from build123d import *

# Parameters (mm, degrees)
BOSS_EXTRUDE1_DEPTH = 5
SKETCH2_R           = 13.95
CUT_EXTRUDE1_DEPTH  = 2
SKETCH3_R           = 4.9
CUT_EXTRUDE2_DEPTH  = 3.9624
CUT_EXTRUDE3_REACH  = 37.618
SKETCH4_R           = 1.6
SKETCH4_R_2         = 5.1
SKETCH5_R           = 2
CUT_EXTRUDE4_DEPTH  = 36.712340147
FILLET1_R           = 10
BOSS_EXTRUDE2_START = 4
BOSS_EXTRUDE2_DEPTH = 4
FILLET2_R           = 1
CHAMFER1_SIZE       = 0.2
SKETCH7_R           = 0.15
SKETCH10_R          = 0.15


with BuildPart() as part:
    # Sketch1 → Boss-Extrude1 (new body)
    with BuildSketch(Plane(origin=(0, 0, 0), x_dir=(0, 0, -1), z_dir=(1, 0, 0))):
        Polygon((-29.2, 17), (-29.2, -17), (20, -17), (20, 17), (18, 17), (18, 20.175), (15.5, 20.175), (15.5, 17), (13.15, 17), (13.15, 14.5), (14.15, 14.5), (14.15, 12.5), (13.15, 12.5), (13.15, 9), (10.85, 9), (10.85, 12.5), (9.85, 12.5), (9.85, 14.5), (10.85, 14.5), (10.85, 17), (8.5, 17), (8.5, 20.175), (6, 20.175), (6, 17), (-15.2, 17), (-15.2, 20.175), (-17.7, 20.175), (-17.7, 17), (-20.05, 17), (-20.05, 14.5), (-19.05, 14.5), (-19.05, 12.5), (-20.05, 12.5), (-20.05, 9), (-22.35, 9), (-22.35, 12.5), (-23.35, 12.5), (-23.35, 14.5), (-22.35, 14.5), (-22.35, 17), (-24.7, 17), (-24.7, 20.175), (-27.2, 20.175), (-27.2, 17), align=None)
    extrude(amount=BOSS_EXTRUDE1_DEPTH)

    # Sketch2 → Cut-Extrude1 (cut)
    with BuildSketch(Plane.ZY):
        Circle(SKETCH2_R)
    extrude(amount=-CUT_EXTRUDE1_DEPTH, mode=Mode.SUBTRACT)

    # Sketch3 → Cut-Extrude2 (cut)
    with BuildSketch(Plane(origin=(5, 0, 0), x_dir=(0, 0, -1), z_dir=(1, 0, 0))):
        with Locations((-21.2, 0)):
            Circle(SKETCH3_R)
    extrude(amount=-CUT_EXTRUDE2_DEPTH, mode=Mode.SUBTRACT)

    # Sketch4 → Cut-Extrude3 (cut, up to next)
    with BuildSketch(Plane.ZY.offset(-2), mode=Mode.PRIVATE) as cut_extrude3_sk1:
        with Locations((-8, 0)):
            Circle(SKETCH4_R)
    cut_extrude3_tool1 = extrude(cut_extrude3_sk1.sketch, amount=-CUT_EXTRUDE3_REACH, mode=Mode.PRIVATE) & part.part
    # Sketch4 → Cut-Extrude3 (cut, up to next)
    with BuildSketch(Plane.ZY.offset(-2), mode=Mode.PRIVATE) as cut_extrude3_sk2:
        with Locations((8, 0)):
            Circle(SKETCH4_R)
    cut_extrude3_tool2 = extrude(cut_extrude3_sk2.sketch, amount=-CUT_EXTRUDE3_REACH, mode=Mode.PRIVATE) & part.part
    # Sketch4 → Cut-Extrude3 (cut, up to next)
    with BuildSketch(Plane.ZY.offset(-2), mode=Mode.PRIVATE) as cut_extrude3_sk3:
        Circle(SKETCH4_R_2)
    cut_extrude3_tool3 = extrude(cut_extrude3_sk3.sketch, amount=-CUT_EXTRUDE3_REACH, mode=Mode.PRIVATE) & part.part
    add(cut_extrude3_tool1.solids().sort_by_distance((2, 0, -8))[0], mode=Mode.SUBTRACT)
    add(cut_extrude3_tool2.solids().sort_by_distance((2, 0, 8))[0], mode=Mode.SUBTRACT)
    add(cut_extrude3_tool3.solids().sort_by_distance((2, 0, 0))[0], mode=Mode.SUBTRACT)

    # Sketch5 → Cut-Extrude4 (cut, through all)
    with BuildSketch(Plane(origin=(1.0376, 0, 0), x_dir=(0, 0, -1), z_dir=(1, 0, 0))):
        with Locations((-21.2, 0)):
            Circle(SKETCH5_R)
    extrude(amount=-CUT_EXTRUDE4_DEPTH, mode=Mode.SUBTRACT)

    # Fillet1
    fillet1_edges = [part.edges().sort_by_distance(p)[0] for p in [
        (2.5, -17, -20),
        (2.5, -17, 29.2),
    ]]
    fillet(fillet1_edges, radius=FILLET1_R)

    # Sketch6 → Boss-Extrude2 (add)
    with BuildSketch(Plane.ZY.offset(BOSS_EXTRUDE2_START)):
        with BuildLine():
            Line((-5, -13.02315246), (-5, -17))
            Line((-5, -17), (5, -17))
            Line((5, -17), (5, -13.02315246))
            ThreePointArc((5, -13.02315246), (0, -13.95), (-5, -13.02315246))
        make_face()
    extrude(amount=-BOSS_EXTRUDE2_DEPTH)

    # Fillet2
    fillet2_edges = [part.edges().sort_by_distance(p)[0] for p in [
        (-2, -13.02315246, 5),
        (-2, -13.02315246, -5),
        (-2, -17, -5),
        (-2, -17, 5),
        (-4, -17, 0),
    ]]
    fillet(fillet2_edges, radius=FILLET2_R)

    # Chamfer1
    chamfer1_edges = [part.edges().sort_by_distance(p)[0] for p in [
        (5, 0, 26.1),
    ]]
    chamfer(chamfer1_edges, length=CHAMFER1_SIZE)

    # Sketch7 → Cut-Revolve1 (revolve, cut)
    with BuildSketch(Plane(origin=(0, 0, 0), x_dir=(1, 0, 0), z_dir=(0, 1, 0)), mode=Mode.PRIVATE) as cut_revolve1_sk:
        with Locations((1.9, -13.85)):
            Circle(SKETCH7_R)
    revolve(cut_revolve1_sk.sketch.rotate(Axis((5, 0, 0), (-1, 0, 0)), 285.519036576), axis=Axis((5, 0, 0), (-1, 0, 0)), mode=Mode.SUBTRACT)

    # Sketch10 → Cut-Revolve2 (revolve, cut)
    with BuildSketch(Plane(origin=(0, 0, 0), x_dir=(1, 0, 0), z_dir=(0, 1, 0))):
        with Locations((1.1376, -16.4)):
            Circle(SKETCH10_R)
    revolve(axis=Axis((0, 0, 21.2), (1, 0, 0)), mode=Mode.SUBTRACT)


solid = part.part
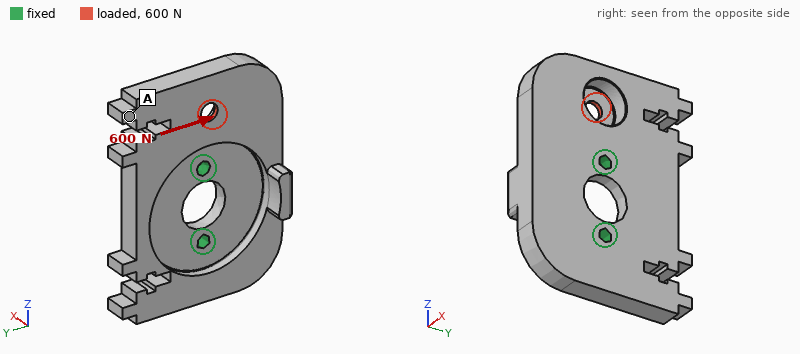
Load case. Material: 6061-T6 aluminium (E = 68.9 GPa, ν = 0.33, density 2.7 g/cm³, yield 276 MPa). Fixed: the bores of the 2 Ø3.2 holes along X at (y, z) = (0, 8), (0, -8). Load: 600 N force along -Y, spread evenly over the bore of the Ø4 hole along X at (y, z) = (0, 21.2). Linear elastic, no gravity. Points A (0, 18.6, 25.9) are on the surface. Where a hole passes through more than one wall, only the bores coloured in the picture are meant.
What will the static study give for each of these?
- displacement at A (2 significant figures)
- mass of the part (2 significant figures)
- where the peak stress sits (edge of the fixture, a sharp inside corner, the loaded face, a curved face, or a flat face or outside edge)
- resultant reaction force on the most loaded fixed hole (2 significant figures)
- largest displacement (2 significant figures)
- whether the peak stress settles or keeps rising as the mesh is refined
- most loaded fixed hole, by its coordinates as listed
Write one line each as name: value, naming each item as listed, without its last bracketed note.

displacement at A: 44 µm
mass of the part: 17 g
where the peak stress sits: edge of the fixture
resultant reaction force on the most loaded fixed hole: 970 N
largest displacement: 48 µm
whether the peak stress settles or keeps rising as the mesh is refined: keeps rising
most loaded fixed hole, by its coordinates as listed: (0, 8)
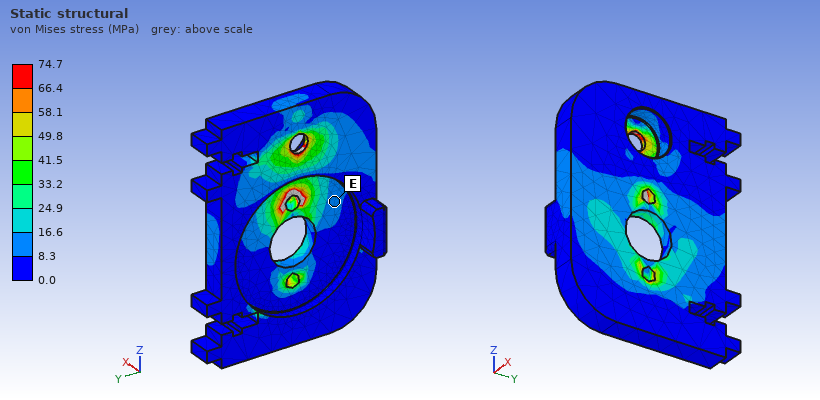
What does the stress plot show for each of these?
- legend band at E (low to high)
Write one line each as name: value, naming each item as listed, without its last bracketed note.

legend band at E: 8.3 to 16.6 MPa
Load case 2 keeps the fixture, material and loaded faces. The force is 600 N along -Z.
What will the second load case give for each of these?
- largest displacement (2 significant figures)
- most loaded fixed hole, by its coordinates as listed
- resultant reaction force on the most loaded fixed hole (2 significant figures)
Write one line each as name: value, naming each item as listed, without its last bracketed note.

largest displacement: 37 µm
most loaded fixed hole, by its coordinates as listed: (0, 8)
resultant reaction force on the most loaded fixed hole: 440 N
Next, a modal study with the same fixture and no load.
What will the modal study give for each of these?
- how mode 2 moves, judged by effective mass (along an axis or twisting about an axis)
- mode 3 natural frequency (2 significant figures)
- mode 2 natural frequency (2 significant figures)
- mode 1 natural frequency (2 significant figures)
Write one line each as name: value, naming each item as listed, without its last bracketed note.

how mode 2 moves, judged by effective mass: along X
mode 3 natural frequency: 7400 Hz
mode 2 natural frequency: 5000 Hz
mode 1 natural frequency: 4500 Hz
